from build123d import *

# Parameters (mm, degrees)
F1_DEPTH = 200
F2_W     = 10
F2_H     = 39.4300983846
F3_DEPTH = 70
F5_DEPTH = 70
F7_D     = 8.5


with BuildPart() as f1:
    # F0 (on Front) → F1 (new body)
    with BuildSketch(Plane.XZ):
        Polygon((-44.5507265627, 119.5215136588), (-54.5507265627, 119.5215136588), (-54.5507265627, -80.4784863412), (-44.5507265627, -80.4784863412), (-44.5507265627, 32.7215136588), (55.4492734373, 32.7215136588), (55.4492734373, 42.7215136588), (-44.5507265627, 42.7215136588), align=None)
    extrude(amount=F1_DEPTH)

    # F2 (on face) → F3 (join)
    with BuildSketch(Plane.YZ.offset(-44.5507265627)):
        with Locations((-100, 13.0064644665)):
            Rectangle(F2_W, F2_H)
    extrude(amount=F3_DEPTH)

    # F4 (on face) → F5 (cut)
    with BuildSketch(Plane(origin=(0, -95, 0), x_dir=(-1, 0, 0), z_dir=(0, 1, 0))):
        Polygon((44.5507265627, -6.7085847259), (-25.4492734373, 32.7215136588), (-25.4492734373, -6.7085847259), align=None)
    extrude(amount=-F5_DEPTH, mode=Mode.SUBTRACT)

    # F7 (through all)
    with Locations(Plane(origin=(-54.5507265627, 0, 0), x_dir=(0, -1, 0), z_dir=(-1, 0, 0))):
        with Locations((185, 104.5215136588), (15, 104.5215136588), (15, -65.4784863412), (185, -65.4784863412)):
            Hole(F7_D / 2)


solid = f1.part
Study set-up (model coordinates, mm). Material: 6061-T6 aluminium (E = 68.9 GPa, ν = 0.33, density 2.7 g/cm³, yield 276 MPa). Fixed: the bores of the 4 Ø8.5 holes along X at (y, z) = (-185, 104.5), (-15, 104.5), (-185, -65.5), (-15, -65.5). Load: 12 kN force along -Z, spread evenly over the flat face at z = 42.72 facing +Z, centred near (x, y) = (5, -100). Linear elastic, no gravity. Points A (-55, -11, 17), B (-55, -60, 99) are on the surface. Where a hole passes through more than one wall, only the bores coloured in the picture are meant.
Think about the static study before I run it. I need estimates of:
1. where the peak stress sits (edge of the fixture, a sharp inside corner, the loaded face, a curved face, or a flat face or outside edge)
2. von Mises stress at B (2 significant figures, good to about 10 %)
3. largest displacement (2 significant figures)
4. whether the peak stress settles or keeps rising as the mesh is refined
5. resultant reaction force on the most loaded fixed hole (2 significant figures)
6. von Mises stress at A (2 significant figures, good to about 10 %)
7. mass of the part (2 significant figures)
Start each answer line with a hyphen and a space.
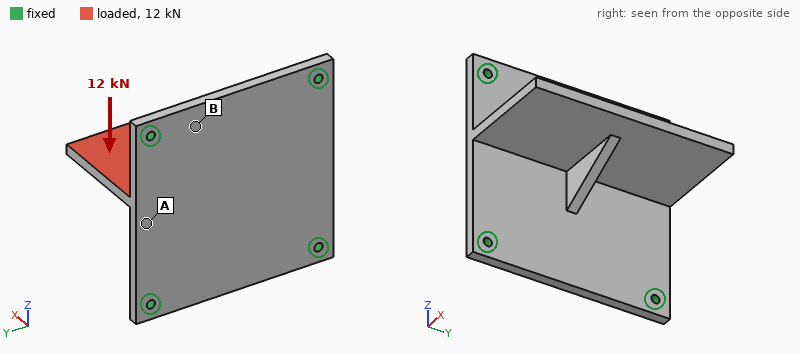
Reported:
- edge of the fixture
- 13 MPa
- 1.2 mm
- keeps rising
- 4.2 kN
- 41 MPa
- 1.7 kg
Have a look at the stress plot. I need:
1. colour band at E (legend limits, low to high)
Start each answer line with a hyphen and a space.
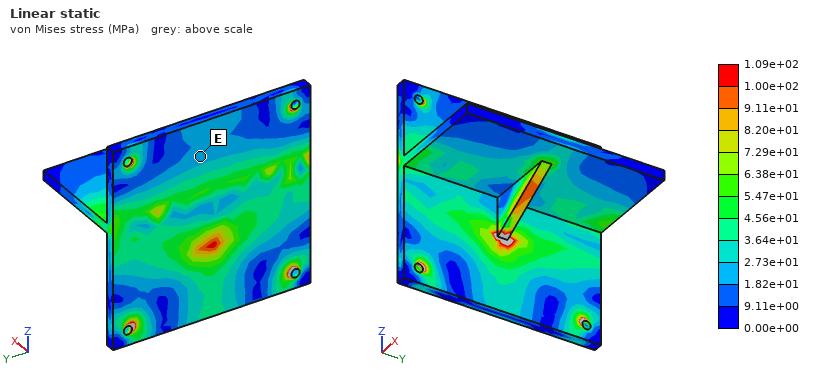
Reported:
- 1.82e+01 to 2.73e+01 MPa
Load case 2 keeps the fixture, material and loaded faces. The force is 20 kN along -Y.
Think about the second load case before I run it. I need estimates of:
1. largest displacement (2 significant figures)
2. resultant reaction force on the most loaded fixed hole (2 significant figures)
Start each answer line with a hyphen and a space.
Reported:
- 0.83 mm
- 7.9 kN
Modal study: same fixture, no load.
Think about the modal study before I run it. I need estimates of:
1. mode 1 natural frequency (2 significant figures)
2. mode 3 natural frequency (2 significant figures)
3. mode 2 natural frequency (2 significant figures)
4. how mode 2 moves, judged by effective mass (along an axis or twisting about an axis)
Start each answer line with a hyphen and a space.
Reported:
- 820 Hz
- 990 Hz
- 950 Hz
- along X
